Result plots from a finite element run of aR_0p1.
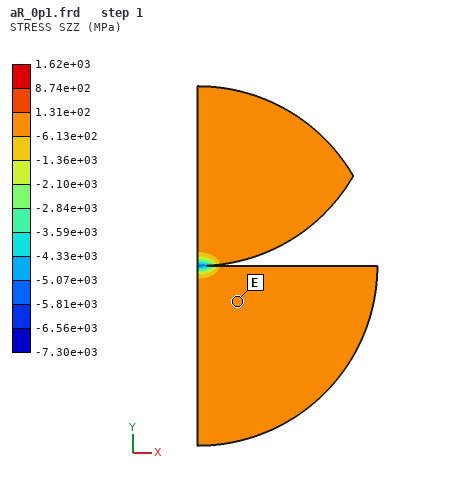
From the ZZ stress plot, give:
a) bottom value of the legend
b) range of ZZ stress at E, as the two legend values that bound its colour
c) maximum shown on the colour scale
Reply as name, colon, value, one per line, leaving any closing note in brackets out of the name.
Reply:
bottom value of the legend: -7.30e+03 MPa
range of ZZ stress at E, as the two legend values that bound its colour: -6.13e+02 to 1.31e+02 MPa
maximum shown on the colour scale: 1.62e+03 MPa
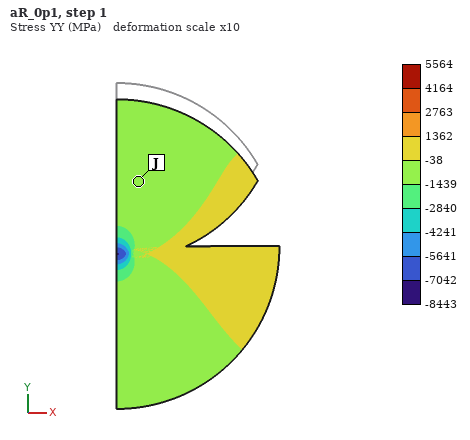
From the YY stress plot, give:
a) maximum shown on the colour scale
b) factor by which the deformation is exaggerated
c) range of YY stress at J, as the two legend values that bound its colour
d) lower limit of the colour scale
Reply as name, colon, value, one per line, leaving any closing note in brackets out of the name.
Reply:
maximum shown on the colour scale: 5564 MPa
factor by which the deformation is exaggerated: 10
range of YY stress at J, as the two legend values that bound its colour: -1439 to -38 MPa
lower limit of the colour scale: -8443 MPa
